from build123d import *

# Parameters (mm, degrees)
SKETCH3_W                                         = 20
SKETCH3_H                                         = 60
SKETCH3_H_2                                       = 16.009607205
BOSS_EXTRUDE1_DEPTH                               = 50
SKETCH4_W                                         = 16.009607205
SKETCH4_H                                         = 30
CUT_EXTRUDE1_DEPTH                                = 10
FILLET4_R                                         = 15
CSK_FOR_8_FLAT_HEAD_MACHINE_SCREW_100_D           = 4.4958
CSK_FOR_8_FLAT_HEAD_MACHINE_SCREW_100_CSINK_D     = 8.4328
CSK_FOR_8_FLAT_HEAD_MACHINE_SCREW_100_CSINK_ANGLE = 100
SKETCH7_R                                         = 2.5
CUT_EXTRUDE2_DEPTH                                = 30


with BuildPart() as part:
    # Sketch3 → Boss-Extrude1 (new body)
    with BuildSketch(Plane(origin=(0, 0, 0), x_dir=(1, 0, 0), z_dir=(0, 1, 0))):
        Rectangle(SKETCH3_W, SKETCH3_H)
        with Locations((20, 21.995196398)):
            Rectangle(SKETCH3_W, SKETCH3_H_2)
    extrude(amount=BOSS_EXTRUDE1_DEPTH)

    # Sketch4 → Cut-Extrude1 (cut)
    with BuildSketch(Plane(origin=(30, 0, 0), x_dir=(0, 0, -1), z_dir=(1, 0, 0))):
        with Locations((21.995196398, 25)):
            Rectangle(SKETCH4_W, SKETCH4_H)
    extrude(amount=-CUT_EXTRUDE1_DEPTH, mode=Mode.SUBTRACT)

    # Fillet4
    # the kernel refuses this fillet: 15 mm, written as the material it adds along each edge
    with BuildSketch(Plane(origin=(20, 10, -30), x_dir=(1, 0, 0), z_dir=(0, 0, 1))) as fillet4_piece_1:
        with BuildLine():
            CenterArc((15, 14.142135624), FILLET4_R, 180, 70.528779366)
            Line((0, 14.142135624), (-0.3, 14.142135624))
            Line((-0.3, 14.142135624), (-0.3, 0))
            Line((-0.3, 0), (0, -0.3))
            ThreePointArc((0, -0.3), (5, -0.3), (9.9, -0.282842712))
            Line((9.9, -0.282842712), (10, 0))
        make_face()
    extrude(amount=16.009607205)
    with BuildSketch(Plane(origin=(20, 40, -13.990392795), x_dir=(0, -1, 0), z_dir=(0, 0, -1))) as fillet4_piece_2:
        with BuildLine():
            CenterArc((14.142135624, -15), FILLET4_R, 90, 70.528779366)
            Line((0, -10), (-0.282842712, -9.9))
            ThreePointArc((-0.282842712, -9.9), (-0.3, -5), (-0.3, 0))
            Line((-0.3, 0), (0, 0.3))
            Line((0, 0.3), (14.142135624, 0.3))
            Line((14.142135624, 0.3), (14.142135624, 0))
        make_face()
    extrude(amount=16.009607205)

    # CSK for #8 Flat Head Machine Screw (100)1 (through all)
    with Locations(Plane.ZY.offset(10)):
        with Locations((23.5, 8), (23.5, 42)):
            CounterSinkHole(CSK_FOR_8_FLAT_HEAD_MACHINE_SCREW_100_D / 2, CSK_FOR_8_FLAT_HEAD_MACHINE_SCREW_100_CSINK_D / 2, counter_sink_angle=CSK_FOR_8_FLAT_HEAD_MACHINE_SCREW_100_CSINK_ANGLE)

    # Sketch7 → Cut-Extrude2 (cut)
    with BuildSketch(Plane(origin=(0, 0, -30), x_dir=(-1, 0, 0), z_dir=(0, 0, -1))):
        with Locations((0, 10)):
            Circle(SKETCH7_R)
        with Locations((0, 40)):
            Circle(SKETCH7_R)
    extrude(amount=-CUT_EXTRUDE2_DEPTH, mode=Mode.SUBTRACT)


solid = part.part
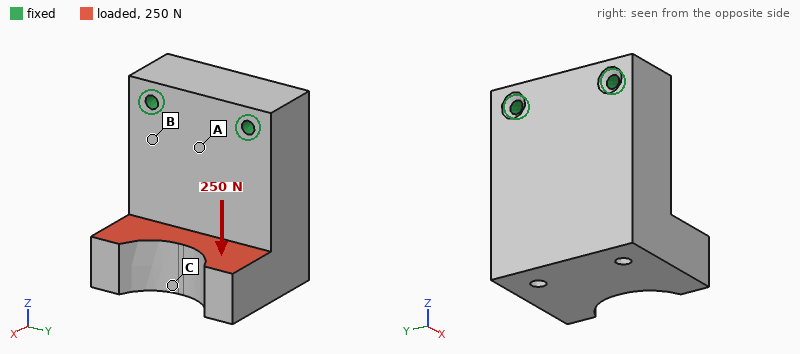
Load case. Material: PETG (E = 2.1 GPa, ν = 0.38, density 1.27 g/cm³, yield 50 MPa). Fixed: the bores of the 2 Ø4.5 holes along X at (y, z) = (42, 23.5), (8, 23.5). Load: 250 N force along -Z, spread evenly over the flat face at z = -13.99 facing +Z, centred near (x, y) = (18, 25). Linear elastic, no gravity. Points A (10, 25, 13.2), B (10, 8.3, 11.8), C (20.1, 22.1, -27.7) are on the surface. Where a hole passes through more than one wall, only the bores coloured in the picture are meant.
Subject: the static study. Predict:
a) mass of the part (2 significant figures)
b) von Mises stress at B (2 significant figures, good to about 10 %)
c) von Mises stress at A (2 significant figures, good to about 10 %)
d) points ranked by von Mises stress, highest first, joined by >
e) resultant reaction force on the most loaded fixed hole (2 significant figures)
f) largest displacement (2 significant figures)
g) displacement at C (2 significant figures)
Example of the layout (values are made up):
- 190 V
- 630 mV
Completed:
- 90 g
- 2.0 MPa
- 0.99 MPa
- B > A > C
- 130 N
- 0.17 mm
- 0.13 mm
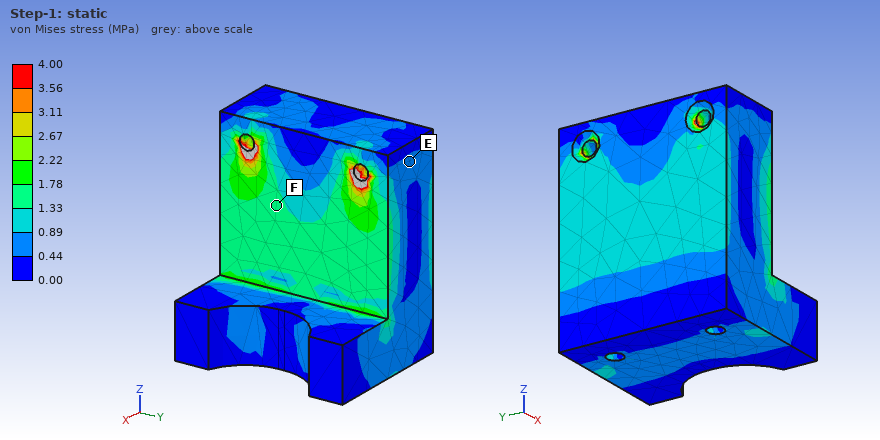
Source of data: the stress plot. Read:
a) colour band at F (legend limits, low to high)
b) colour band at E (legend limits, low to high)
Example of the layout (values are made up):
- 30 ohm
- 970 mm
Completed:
- 1.33 to 1.78 MPa
- 0.44 to 0.89 MPa
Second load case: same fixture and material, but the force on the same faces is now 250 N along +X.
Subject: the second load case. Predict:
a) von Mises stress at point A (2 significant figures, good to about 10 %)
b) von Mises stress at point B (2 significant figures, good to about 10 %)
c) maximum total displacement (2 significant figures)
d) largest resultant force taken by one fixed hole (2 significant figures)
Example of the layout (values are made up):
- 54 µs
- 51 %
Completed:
- 1.1 MPa
- 2.5 MPa
- 0.19 mm
- 130 N
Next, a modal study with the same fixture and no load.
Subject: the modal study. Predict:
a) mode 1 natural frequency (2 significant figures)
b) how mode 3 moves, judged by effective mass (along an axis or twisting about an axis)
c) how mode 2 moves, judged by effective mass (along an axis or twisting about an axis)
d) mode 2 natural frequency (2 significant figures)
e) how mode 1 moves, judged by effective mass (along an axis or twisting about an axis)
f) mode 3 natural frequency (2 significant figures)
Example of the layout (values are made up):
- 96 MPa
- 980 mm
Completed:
- 850 Hz
- along Y
- along Y
- 1600 Hz
- along X
- 2100 Hz
